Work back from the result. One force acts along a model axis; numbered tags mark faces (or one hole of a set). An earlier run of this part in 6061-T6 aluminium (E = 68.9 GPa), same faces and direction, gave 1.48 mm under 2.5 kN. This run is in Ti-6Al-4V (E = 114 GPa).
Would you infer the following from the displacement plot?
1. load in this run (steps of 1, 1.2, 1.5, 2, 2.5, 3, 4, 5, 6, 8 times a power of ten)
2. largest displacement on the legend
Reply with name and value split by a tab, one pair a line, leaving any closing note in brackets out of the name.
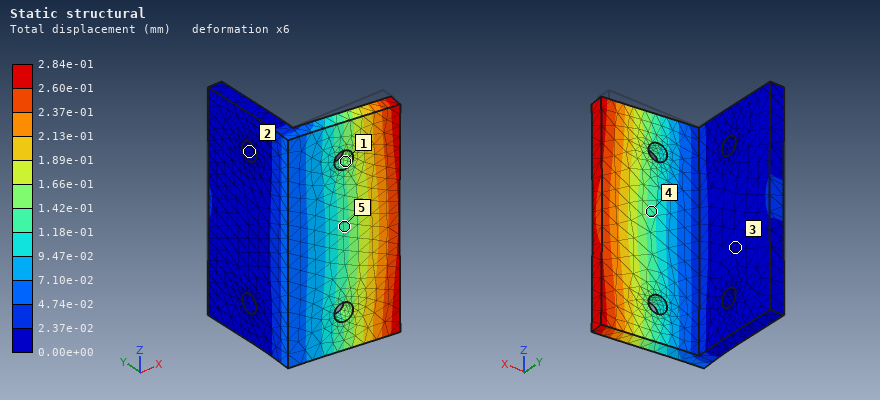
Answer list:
load in this run	800 N
largest displacement on the legend	2.84e-01 mm
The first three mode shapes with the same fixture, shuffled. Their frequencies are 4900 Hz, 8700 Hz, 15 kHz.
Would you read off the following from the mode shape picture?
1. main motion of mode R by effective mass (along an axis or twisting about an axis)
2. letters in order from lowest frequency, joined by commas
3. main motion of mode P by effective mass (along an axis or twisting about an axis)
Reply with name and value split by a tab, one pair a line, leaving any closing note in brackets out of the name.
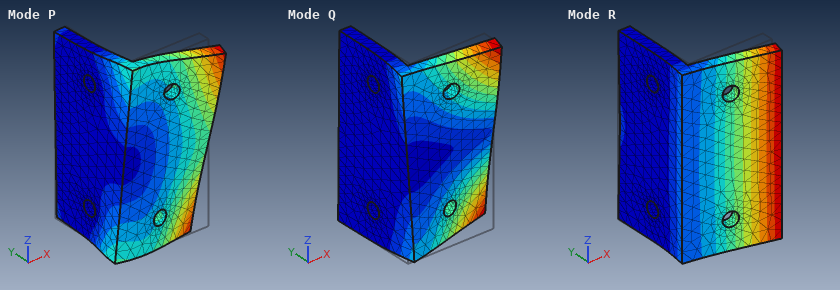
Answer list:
main motion of mode R by effective mass	along Y
letters in order from lowest frequency, joined by commas	R, Q, P
main motion of mode P by effective mass	along Z
